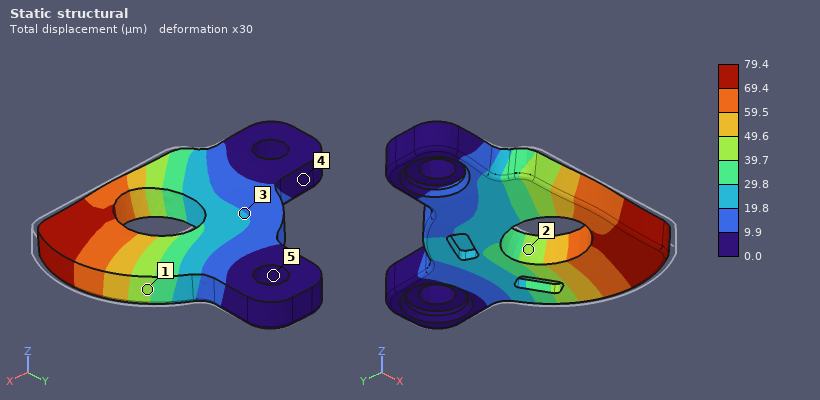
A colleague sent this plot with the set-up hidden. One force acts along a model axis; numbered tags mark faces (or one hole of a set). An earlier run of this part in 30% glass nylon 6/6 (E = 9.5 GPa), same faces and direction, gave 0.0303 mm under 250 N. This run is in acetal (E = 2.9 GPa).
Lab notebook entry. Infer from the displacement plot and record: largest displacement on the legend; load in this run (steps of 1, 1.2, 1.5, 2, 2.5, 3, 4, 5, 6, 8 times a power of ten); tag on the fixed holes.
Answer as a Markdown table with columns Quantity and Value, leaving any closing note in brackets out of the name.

| Quantity | Value |
|---|---|
| largest displacement on the legend | 79.4 µm |
| load in this run | 200 N |
| tag on the fixed holes | 5 |
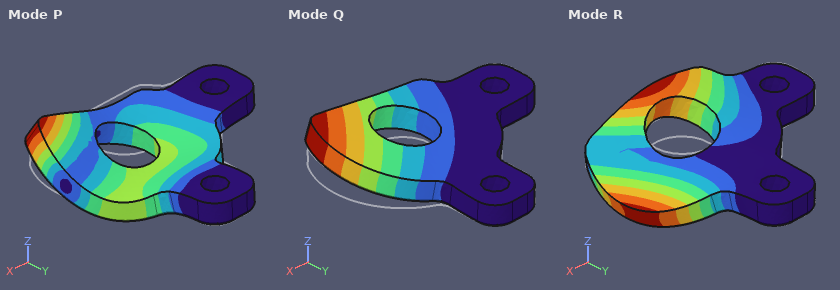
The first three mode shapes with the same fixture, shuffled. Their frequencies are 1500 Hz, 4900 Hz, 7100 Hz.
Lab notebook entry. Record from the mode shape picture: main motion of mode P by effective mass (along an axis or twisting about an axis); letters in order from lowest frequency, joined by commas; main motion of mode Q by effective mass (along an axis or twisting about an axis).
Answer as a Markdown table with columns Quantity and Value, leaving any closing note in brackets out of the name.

| Quantity | Value |
|---|---|
| main motion of mode P by effective mass | along Z |
| letters in order from lowest frequency, joined by commas | Q, R, P |
| main motion of mode Q by effective mass | along Z |
